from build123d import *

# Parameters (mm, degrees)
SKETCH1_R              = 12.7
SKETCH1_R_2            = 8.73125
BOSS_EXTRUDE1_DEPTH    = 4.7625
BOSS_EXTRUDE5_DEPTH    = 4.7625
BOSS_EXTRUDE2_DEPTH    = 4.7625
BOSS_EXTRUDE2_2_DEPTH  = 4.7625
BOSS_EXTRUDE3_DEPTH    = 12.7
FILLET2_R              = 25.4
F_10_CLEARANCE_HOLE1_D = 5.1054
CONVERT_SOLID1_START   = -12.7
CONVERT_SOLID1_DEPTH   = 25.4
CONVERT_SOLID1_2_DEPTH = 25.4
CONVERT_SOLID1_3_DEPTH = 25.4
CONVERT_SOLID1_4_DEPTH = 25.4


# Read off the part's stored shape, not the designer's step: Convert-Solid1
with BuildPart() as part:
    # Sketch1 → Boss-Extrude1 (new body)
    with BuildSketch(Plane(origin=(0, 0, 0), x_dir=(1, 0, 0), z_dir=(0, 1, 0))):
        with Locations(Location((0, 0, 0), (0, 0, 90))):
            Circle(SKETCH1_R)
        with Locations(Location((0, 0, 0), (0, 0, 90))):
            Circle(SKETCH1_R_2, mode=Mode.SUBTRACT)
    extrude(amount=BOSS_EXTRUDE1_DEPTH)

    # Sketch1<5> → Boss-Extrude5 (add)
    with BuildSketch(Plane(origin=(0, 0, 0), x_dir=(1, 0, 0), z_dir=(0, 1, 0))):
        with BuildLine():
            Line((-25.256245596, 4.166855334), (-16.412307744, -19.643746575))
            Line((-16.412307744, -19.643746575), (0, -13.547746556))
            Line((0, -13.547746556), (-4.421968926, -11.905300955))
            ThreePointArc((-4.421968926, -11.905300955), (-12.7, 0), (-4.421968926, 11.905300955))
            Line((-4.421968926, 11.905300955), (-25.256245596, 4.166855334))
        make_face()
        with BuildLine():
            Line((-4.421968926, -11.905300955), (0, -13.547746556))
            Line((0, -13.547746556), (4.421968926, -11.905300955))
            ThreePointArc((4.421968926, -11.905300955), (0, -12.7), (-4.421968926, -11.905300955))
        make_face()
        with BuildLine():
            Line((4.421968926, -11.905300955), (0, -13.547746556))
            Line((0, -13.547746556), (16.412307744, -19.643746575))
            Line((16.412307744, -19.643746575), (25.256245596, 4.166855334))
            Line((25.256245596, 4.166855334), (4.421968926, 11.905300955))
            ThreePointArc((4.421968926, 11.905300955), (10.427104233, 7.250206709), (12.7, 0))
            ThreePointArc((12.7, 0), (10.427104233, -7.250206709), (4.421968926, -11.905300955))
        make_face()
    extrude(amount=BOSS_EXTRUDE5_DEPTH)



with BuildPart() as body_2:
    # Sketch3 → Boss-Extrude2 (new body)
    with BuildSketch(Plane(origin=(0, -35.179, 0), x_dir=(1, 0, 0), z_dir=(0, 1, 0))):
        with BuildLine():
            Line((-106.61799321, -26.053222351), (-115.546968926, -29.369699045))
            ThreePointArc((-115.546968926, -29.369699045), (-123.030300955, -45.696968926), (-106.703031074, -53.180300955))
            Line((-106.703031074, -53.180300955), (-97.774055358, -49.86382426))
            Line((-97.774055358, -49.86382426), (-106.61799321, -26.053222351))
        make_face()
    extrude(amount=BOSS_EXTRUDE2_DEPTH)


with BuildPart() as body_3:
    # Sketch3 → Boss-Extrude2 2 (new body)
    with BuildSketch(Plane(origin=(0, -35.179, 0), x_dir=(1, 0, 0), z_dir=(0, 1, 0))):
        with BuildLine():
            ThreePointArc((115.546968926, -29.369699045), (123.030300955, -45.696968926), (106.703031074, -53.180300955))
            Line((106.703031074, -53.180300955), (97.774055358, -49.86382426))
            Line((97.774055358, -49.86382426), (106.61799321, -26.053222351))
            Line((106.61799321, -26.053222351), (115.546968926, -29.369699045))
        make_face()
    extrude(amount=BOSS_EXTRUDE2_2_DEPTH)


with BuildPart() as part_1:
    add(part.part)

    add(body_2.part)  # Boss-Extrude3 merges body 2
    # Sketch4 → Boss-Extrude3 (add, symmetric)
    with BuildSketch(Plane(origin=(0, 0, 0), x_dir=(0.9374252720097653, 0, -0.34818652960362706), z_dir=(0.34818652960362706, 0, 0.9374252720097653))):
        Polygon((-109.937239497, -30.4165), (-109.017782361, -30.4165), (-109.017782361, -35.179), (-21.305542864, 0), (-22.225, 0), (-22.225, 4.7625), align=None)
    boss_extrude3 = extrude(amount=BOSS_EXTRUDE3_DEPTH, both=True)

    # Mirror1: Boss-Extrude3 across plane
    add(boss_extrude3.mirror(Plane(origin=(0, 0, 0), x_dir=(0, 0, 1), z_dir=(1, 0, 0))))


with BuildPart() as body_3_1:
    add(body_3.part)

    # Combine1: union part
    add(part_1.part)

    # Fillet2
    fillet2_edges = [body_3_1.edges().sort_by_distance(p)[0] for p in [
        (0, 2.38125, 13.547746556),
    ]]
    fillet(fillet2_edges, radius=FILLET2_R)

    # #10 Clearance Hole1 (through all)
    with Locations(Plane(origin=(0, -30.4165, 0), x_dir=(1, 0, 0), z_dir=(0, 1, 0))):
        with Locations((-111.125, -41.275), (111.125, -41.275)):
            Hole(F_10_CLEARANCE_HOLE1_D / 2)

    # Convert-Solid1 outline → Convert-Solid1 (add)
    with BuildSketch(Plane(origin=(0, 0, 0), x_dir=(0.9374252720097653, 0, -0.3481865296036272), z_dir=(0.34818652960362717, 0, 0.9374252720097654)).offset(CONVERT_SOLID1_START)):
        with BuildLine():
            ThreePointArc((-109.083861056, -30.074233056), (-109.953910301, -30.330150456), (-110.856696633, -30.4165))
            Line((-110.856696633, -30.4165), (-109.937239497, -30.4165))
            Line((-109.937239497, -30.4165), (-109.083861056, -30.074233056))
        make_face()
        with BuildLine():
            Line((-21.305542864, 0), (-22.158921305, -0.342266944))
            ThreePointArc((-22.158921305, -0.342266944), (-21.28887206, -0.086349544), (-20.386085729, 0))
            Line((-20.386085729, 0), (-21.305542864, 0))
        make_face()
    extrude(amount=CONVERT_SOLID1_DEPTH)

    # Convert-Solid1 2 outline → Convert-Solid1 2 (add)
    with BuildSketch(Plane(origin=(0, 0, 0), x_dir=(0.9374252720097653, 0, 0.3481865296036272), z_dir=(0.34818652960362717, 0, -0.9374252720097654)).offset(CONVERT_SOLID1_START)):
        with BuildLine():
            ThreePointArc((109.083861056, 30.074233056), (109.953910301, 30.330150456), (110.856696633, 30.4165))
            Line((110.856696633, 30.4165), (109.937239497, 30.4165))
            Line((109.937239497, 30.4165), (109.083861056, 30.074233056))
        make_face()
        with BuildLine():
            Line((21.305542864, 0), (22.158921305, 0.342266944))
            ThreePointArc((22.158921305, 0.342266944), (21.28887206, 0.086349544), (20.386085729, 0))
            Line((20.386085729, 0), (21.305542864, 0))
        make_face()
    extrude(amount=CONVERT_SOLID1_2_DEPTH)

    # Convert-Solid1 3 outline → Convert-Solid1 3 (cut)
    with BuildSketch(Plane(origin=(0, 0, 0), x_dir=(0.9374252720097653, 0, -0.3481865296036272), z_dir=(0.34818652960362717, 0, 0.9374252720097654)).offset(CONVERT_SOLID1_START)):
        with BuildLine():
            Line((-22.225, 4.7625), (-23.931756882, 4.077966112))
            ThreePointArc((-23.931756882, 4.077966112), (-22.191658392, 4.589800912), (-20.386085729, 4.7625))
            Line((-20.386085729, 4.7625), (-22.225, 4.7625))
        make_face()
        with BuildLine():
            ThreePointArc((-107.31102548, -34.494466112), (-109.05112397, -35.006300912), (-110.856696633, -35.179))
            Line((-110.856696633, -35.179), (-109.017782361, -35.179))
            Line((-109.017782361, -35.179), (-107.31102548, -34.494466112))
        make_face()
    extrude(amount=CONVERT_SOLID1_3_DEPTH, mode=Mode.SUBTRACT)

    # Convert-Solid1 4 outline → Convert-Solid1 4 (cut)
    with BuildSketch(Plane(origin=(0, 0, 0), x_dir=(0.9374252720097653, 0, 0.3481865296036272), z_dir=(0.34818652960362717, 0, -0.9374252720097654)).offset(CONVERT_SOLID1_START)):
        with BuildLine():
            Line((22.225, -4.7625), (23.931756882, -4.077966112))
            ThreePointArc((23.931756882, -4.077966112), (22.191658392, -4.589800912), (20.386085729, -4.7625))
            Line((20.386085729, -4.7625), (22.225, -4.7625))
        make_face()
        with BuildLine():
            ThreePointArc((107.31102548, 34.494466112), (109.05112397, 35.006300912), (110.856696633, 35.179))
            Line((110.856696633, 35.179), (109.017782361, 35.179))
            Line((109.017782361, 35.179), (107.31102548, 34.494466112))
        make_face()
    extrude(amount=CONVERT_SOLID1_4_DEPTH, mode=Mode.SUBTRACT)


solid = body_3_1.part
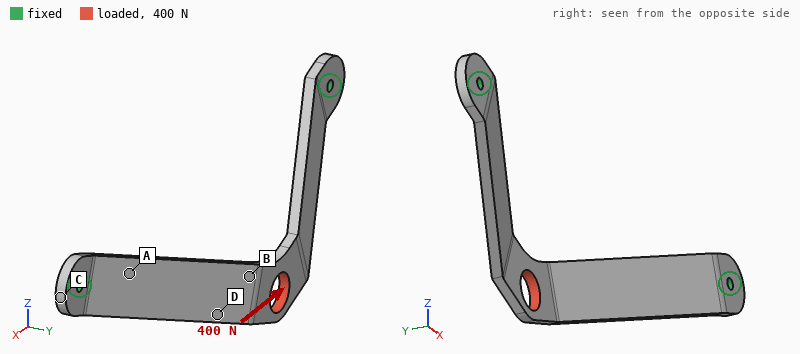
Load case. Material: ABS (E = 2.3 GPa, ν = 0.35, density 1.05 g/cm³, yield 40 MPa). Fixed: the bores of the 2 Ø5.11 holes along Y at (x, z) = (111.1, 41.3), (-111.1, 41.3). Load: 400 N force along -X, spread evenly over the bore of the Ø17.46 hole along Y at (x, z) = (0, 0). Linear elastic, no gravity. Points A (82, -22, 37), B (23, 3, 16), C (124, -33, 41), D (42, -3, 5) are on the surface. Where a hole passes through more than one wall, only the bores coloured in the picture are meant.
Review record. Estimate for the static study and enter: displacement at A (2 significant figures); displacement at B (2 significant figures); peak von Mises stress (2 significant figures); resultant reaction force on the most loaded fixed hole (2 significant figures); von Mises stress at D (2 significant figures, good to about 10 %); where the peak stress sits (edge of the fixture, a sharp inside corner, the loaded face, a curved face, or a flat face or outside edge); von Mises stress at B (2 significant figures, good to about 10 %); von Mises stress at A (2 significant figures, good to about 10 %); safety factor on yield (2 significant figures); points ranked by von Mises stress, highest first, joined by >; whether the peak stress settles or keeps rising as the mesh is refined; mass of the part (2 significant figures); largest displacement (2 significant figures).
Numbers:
0.43 mm
1.4 mm
18 MPa
220 N
7.5 MPa
a curved face
10 MPa
4.8 MPa
2.2
B > D > A > C
settles
33 g
2.1 mm
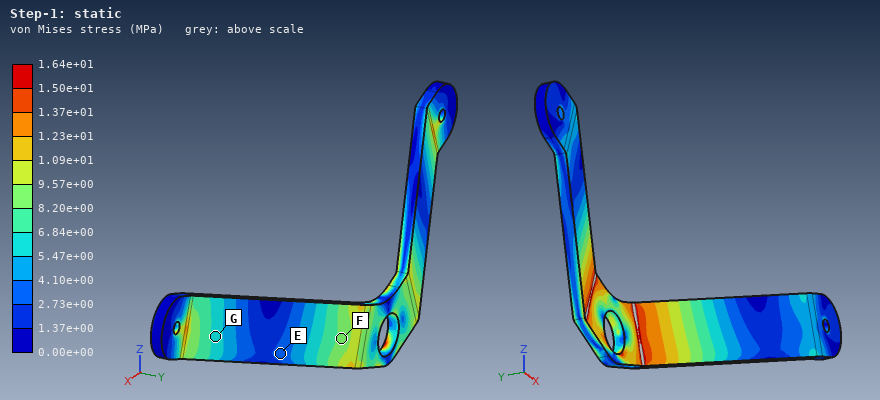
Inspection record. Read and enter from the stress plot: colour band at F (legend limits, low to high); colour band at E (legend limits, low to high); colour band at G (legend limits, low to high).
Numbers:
8.20e+00 to 9.57e+00 MPa
2.73e+00 to 4.10e+00 MPa
5.47e+00 to 6.84e+00 MPa
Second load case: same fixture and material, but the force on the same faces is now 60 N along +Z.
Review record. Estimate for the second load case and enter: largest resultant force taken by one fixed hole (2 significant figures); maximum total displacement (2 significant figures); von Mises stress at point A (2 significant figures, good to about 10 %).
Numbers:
30 N
3.0 mm
4.3 MPa
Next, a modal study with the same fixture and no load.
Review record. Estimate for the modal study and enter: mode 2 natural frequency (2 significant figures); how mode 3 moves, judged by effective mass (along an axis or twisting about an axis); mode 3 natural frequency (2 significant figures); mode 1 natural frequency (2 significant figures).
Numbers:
320 Hz
along Y
530 Hz
200 Hz
